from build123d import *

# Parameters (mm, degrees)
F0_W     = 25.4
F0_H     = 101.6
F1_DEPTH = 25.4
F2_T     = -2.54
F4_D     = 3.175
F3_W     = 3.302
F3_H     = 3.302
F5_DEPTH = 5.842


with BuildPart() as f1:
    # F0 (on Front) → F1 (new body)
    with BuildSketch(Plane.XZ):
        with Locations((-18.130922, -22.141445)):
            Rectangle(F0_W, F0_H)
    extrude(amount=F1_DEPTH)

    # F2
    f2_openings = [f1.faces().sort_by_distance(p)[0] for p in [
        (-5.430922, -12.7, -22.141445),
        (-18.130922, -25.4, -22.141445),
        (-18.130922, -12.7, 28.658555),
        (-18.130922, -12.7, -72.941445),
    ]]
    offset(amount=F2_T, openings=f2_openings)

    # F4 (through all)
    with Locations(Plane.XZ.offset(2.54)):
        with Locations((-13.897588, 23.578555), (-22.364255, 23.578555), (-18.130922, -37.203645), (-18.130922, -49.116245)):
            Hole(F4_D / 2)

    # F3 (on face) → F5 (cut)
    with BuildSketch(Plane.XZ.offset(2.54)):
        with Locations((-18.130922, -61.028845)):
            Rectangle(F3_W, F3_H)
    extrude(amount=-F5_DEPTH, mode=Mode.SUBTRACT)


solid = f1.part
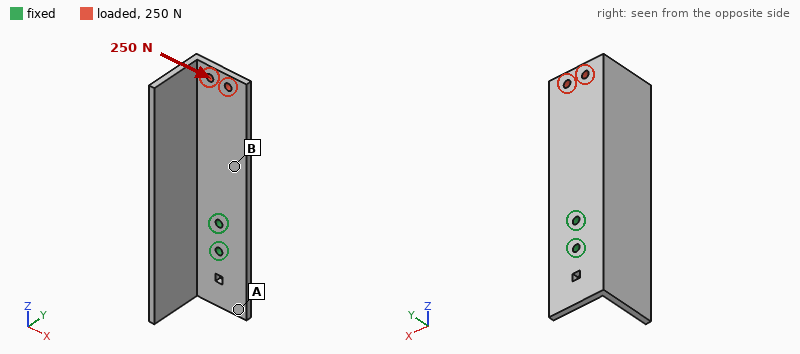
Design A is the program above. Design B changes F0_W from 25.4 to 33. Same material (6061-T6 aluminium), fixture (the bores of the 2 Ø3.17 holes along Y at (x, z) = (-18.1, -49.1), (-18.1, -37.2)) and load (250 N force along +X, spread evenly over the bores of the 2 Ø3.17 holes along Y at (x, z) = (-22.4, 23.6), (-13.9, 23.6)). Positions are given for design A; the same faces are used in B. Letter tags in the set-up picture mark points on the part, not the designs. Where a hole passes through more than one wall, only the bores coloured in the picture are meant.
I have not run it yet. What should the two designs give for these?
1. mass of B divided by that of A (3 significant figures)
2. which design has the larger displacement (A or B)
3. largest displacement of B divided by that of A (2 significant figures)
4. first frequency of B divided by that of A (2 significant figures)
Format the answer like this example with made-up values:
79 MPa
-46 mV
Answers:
1.16
A
0.69
0.82
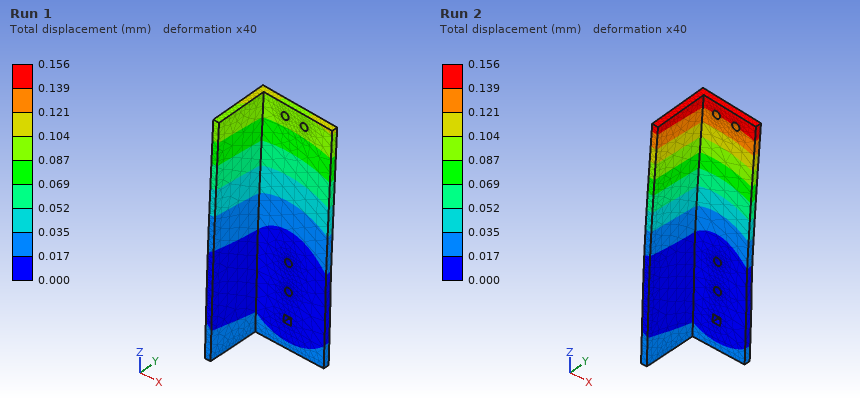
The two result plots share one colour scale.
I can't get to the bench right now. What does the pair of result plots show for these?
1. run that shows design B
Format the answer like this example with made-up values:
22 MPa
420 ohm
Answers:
Run 1
